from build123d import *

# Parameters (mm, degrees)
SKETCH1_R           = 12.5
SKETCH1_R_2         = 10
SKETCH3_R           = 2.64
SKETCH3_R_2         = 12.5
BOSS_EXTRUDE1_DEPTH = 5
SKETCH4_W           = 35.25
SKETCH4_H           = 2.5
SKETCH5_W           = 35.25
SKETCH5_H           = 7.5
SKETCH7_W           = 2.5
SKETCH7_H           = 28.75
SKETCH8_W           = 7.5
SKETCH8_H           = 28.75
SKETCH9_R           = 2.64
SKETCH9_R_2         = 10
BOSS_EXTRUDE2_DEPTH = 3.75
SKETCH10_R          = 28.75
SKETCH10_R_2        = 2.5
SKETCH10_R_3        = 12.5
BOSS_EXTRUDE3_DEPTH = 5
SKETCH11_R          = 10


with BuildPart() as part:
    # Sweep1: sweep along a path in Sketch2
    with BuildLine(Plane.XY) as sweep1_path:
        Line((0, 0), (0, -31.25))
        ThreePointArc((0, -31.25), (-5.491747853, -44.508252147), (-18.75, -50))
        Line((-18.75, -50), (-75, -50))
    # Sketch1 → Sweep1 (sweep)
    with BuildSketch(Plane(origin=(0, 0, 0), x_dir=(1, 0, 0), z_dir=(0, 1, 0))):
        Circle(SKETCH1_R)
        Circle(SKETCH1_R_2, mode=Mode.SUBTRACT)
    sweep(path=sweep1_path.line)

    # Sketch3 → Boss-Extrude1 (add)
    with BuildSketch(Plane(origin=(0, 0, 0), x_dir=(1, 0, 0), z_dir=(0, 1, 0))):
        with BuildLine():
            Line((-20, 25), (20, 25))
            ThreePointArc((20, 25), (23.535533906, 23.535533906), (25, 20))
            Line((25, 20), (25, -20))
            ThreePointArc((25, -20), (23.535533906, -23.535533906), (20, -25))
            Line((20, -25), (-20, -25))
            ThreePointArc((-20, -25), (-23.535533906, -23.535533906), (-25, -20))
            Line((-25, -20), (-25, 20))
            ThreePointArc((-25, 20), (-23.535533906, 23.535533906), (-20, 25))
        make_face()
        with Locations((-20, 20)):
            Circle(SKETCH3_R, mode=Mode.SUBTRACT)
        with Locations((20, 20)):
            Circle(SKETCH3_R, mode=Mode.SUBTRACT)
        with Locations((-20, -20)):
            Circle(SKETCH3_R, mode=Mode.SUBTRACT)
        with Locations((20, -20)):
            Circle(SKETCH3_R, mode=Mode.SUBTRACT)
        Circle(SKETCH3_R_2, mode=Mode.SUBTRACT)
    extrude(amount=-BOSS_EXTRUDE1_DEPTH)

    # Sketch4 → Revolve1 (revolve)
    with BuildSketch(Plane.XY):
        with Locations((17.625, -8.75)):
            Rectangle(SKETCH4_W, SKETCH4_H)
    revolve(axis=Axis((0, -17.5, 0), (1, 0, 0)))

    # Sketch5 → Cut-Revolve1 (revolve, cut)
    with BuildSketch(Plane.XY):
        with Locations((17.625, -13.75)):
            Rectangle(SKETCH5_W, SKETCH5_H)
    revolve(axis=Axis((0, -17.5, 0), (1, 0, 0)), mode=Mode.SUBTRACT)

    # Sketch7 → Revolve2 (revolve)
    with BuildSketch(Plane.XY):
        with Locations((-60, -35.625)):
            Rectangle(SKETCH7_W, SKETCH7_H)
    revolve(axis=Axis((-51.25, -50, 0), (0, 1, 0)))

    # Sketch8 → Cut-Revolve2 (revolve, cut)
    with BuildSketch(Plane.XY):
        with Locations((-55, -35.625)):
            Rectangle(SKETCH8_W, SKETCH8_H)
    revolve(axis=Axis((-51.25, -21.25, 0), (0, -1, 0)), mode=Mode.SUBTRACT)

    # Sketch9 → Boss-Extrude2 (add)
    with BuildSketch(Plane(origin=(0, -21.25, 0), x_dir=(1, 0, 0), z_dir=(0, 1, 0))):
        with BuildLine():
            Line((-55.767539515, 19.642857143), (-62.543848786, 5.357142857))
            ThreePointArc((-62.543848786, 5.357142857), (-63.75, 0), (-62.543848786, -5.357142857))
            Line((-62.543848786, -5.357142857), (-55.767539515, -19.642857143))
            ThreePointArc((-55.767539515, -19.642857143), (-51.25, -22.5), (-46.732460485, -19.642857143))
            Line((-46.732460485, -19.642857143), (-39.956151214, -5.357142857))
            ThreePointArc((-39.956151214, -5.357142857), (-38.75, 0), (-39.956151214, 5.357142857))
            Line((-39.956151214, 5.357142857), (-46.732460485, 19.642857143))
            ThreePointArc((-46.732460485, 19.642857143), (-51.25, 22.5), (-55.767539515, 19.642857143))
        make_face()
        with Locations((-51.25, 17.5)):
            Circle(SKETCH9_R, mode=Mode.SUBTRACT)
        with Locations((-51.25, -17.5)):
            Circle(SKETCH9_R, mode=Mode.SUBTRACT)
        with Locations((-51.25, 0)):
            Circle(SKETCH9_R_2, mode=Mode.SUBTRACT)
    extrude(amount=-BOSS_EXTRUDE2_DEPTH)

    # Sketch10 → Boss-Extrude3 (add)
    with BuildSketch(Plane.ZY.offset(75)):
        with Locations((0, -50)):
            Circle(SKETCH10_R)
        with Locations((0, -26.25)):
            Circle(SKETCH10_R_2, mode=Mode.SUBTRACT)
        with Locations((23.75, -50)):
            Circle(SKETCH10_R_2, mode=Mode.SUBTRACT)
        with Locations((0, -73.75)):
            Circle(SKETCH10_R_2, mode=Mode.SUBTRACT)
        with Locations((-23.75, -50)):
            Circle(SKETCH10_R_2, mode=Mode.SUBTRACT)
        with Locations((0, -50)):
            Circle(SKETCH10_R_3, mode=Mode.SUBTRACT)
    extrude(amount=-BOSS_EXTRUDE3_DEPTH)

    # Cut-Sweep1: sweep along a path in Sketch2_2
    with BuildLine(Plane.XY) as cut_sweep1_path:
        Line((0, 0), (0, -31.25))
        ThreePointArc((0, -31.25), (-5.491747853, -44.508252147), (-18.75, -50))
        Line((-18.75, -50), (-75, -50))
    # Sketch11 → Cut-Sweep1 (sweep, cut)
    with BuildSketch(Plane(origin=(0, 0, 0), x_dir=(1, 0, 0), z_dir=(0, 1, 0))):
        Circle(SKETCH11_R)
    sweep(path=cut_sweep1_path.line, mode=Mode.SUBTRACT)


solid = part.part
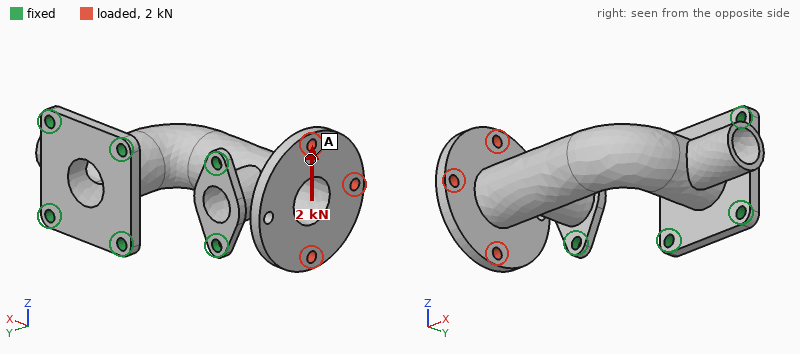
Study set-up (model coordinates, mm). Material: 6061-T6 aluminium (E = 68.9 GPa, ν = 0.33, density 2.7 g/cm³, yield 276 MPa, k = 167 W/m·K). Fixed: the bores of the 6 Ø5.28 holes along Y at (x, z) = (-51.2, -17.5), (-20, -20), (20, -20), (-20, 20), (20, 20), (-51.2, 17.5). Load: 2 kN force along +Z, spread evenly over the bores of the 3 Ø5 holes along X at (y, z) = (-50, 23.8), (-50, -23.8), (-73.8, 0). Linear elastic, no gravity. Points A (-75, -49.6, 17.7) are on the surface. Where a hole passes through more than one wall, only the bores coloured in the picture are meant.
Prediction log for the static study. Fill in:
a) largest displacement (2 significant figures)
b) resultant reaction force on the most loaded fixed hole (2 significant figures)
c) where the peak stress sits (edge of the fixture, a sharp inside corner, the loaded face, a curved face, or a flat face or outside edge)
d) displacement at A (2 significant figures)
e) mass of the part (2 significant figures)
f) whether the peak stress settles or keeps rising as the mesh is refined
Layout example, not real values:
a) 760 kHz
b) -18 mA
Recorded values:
a) 0.43 mm
b) 2.3 kN
c) edge of the fixture
d) 0.26 mm
e) 130 g
f) keeps rising
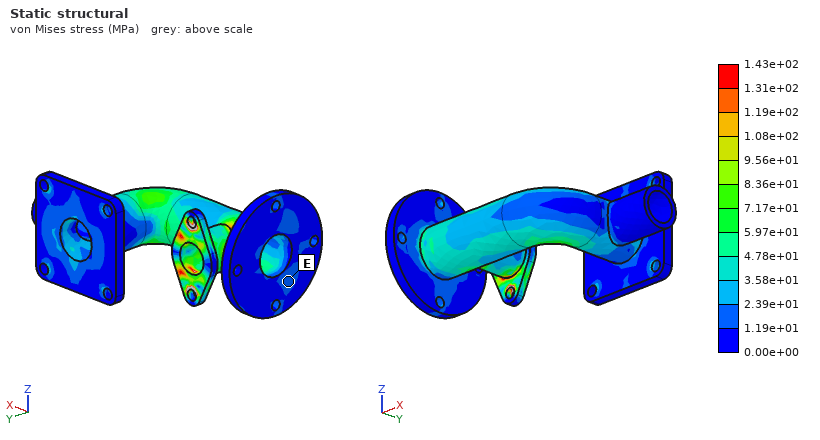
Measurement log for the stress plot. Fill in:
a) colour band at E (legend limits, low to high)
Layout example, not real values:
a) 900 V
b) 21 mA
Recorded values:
a) 1.19e+01 to 2.39e+01 MPa
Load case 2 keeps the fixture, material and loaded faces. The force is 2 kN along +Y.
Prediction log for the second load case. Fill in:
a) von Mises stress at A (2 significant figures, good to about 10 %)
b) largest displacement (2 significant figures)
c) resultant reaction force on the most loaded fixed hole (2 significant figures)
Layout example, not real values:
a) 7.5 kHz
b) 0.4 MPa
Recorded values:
a) 14 MPa
b) 0.16 mm
c) 1.5 kN
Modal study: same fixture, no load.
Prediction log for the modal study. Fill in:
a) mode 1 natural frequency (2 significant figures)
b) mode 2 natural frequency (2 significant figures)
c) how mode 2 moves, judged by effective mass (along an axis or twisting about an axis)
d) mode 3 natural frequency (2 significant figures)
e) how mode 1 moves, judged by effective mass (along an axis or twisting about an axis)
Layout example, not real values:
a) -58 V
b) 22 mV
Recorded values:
a) 2100 Hz
b) 2700 Hz
c) along X
d) 3400 Hz
e) along Z
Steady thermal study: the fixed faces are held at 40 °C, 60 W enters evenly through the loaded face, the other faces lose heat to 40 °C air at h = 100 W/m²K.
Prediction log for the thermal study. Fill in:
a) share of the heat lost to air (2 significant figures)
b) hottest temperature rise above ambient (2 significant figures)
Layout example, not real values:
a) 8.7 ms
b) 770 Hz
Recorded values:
a) 73 %
b) 58 K
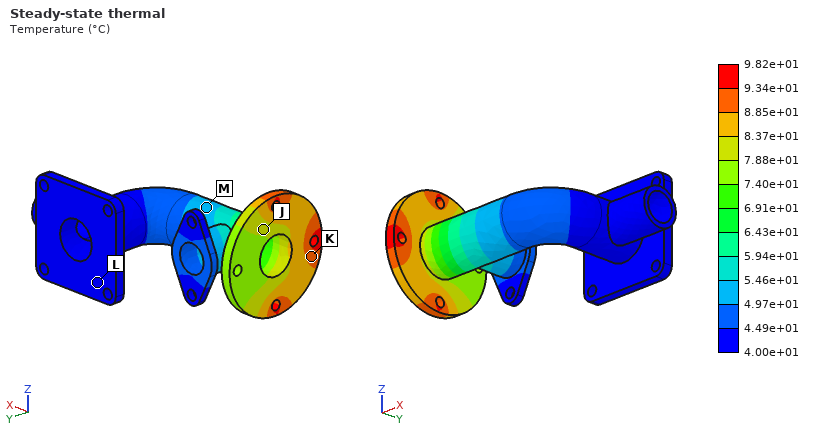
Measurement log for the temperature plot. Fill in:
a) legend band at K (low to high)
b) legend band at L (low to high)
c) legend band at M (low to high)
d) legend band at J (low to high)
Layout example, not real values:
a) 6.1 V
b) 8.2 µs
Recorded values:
a) 8.85e+01 to 9.34e+01 °C
b) 4.00e+01 to 4.49e+01 °C
c) 4.97e+01 to 5.46e+01 °C
d) 7.88e+01 to 8.37e+01 °C
